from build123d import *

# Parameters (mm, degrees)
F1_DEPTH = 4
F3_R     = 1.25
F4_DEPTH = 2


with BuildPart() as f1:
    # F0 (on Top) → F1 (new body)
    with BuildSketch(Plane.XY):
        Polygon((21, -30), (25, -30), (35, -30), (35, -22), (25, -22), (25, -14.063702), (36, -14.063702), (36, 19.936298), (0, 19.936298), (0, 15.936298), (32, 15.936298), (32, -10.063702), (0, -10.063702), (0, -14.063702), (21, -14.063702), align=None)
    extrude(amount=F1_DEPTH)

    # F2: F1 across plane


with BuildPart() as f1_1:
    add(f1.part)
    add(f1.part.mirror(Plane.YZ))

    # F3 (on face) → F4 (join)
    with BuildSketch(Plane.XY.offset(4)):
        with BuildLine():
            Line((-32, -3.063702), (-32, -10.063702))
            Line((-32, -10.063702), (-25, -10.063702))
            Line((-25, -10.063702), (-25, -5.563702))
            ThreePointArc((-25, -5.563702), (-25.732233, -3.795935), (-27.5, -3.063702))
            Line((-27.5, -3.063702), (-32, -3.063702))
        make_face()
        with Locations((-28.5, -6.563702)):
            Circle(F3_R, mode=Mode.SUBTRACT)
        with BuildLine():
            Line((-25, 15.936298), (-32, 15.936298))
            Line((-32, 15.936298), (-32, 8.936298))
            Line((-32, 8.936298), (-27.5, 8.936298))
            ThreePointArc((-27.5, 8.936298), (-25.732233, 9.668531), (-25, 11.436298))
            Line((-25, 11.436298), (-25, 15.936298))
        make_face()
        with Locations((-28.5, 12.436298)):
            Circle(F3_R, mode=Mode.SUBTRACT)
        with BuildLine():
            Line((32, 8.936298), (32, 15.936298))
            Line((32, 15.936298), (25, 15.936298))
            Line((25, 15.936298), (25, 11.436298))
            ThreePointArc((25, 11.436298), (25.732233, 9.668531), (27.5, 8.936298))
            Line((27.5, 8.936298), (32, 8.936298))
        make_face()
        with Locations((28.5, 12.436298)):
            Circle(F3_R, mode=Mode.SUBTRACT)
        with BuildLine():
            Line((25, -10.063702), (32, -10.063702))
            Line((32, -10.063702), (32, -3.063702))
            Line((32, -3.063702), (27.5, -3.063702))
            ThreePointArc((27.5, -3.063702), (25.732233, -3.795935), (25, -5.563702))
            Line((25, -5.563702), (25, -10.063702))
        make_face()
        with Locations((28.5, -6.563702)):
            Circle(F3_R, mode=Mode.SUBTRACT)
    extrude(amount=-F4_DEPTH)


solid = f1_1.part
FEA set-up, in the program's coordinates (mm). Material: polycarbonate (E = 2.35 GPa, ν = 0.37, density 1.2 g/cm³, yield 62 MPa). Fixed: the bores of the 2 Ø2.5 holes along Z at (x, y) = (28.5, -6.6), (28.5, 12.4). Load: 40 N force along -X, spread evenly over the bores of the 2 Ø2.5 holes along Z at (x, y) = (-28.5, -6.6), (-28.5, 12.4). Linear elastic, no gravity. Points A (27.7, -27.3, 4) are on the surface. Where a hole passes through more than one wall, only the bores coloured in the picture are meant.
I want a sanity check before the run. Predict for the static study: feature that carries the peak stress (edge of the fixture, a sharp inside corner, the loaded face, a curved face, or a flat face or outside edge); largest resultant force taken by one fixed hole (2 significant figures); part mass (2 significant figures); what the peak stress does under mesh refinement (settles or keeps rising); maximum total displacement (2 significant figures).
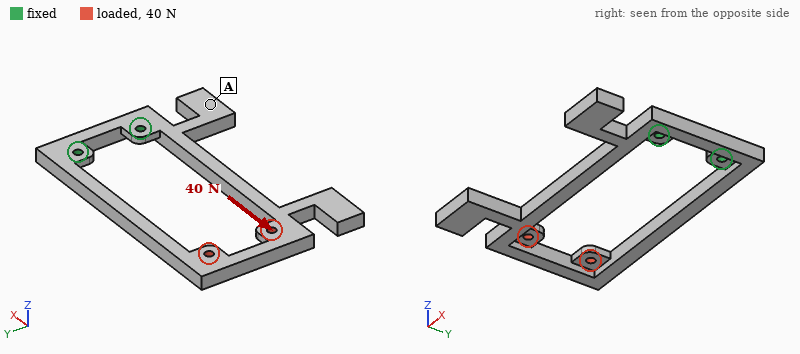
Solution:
edge of the fixture
25 N
5.6 g
keeps rising
0.85 mm
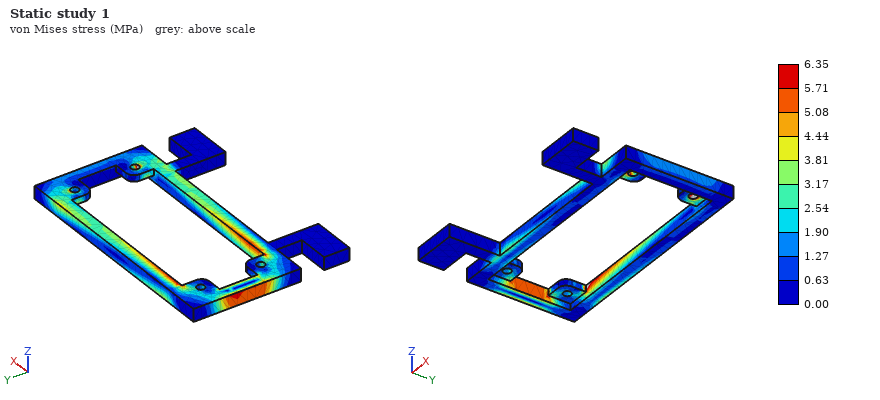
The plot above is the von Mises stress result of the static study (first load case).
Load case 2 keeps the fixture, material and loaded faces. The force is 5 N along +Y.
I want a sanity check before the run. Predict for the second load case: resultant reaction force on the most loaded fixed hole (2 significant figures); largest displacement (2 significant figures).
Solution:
8.7 N
0.96 mm
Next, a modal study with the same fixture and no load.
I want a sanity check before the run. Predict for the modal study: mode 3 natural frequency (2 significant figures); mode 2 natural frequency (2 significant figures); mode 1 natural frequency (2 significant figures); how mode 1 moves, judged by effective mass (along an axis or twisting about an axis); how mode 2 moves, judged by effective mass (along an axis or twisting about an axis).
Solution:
270 Hz
240 Hz
110 Hz
along Z
along Y
